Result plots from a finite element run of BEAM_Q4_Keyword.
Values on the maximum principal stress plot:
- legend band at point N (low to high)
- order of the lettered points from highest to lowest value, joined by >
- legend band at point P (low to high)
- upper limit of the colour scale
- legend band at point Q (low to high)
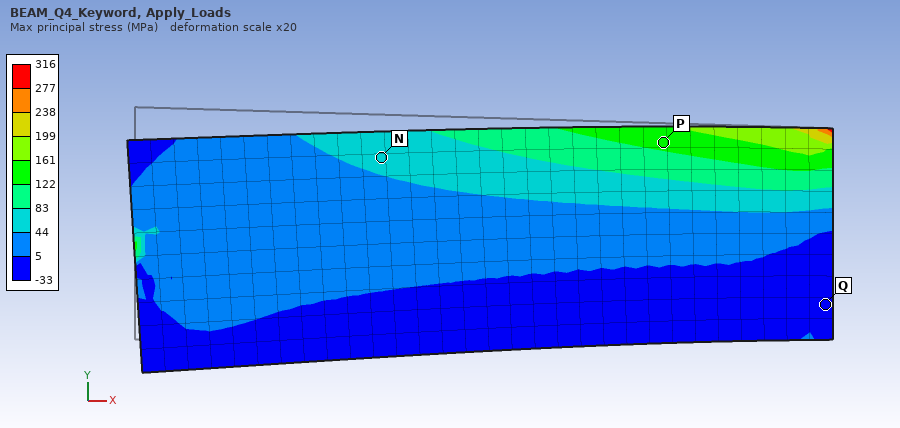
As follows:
44 to 83 MPa
P > N > Q
122 to 161 MPa
316 MPa
-33 to 5 MPa
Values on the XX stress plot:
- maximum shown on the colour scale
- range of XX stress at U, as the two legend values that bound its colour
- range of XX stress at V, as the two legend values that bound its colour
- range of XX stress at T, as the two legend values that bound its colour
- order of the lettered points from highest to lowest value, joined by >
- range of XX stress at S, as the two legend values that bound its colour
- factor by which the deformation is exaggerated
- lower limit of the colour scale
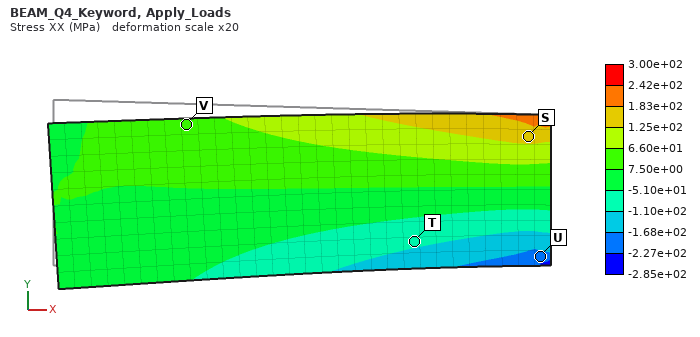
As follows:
3.00e+02 MPa
-2.27e+02 to -1.68e+02 MPa
7.50e+00 to 6.60e+01 MPa
-1.10e+02 to -5.10e+01 MPa
S > V > T > U
1.25e+02 to 1.83e+02 MPa
20
-2.85e+02 MPa
